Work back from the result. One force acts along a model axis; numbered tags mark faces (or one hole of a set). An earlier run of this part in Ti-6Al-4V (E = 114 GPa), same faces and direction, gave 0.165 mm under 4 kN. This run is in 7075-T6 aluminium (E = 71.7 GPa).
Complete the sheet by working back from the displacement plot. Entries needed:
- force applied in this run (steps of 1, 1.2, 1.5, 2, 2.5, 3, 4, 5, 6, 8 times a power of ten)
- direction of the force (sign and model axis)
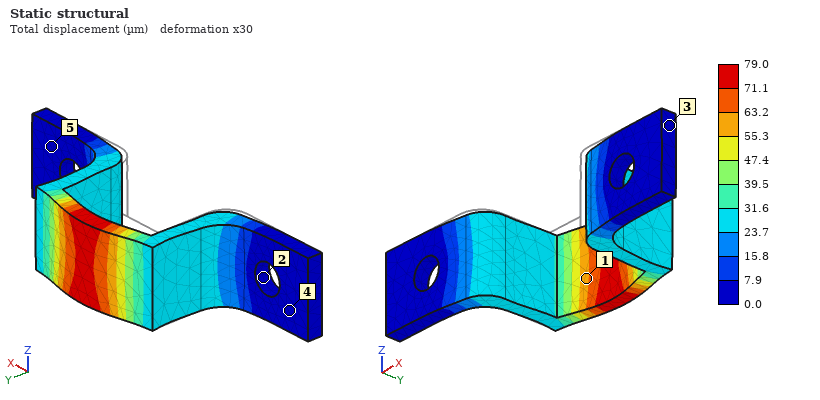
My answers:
1.2 kN
+Y
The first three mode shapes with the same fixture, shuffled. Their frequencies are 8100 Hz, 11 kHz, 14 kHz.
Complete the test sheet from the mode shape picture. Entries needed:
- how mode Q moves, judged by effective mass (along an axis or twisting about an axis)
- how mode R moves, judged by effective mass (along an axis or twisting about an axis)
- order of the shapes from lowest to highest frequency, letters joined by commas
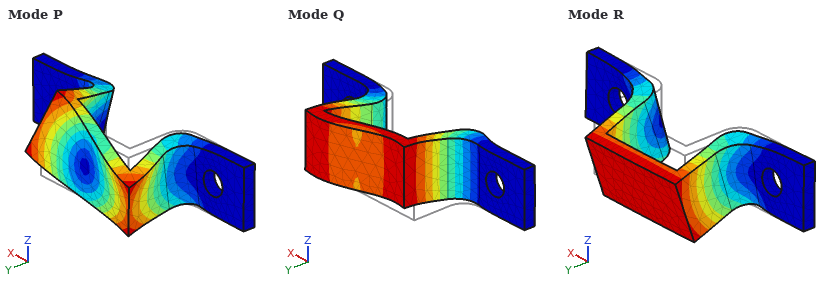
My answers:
along X
along Z
R, Q, P
